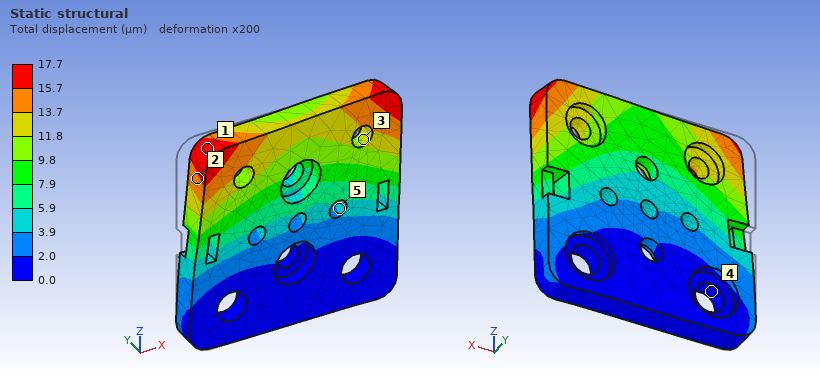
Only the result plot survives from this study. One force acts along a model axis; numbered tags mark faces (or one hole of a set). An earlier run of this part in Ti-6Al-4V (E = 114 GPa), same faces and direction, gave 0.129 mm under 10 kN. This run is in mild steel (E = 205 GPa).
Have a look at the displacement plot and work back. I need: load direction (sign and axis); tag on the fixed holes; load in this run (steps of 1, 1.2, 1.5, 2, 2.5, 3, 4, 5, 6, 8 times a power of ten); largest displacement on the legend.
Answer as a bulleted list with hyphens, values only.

- +X
- 4
- 2.5 kN
- 17.7 µm
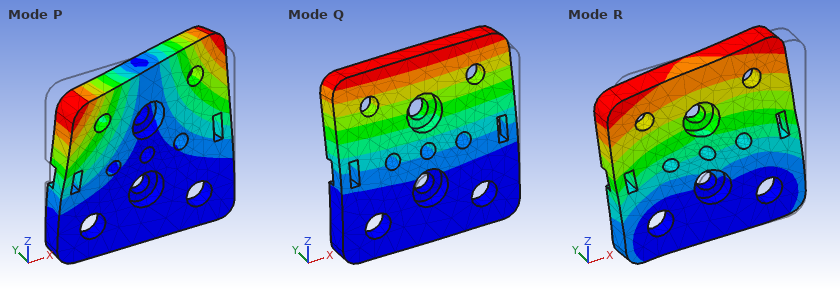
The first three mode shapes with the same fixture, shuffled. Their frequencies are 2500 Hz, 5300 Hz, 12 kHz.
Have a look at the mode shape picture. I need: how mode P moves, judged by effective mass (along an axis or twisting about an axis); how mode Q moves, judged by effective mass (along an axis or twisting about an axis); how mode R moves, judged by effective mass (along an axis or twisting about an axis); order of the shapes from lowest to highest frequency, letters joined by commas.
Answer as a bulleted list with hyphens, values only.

- twisting about Z
- along Y
- along X
- Q, P, R
